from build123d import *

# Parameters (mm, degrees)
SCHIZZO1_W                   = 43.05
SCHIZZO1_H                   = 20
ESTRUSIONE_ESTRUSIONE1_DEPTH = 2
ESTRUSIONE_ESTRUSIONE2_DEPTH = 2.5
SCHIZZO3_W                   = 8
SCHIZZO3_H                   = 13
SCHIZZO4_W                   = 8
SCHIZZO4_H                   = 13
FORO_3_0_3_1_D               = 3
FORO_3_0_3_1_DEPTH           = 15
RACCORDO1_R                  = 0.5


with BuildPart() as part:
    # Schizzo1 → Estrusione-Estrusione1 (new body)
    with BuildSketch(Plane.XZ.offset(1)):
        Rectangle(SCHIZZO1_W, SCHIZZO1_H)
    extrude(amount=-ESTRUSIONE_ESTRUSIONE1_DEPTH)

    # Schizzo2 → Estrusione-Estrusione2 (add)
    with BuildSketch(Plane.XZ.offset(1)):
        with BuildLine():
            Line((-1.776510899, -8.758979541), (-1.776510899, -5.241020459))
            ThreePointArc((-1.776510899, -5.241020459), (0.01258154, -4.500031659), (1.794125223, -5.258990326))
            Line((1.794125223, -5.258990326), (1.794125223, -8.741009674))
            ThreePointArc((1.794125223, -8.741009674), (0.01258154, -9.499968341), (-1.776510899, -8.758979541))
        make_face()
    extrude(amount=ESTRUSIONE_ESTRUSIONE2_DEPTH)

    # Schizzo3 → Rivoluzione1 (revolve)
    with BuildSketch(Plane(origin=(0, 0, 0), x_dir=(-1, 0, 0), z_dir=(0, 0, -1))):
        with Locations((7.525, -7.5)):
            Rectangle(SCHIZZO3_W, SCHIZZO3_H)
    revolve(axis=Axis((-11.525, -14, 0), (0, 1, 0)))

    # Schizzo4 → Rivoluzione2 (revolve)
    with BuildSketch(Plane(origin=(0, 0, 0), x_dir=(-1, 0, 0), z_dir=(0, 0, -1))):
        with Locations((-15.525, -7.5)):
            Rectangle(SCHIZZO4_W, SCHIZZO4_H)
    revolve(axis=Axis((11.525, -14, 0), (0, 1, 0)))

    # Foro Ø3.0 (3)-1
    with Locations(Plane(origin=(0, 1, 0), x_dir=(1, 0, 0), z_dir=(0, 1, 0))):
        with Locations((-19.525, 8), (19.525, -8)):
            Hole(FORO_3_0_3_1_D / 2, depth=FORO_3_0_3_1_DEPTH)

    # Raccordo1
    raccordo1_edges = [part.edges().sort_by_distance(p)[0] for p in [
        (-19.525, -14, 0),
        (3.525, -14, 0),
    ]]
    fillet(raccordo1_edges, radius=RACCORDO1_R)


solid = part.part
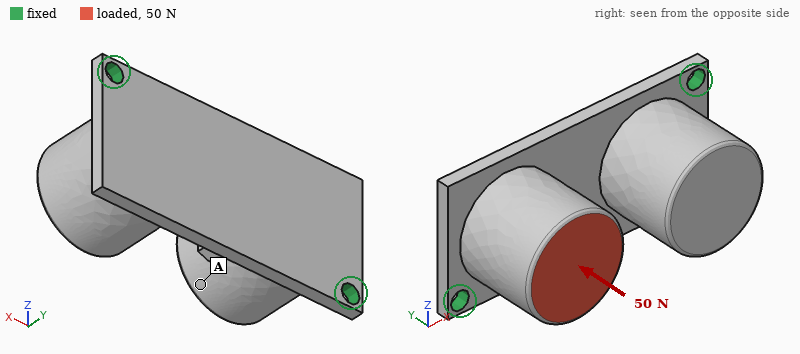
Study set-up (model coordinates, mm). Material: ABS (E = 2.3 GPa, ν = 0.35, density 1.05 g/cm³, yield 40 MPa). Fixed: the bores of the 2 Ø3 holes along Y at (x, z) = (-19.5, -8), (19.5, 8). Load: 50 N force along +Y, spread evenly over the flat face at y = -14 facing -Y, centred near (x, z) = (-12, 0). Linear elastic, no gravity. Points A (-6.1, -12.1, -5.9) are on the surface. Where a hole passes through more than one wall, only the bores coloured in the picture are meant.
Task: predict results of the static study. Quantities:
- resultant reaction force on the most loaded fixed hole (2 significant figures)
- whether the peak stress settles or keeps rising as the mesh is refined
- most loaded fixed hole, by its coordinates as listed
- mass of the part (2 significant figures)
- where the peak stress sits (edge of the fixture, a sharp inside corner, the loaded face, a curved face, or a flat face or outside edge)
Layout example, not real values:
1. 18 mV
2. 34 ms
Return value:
1. 39 N
2. keeps rising
3. (-19.5, -8)
4. 7.3 g
5. edge of the fixture
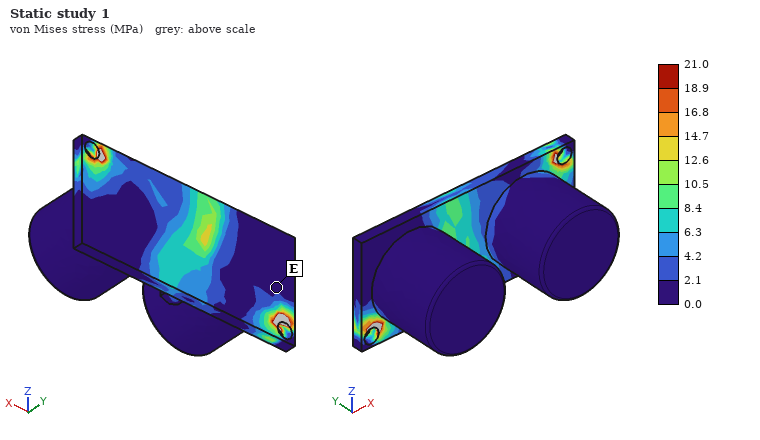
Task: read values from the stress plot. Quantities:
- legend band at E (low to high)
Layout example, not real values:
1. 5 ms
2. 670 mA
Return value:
1. 0.0 to 2.1 MPa
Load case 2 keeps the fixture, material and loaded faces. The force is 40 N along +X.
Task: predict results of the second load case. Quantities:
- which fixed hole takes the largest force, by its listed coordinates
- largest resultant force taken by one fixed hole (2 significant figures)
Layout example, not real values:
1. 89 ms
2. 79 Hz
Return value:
1. (-19.5, -8)
2. 27 N
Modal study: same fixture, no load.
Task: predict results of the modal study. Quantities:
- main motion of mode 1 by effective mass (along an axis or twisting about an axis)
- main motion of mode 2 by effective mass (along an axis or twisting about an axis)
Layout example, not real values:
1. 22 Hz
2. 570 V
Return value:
1. along Z
2. along Y
